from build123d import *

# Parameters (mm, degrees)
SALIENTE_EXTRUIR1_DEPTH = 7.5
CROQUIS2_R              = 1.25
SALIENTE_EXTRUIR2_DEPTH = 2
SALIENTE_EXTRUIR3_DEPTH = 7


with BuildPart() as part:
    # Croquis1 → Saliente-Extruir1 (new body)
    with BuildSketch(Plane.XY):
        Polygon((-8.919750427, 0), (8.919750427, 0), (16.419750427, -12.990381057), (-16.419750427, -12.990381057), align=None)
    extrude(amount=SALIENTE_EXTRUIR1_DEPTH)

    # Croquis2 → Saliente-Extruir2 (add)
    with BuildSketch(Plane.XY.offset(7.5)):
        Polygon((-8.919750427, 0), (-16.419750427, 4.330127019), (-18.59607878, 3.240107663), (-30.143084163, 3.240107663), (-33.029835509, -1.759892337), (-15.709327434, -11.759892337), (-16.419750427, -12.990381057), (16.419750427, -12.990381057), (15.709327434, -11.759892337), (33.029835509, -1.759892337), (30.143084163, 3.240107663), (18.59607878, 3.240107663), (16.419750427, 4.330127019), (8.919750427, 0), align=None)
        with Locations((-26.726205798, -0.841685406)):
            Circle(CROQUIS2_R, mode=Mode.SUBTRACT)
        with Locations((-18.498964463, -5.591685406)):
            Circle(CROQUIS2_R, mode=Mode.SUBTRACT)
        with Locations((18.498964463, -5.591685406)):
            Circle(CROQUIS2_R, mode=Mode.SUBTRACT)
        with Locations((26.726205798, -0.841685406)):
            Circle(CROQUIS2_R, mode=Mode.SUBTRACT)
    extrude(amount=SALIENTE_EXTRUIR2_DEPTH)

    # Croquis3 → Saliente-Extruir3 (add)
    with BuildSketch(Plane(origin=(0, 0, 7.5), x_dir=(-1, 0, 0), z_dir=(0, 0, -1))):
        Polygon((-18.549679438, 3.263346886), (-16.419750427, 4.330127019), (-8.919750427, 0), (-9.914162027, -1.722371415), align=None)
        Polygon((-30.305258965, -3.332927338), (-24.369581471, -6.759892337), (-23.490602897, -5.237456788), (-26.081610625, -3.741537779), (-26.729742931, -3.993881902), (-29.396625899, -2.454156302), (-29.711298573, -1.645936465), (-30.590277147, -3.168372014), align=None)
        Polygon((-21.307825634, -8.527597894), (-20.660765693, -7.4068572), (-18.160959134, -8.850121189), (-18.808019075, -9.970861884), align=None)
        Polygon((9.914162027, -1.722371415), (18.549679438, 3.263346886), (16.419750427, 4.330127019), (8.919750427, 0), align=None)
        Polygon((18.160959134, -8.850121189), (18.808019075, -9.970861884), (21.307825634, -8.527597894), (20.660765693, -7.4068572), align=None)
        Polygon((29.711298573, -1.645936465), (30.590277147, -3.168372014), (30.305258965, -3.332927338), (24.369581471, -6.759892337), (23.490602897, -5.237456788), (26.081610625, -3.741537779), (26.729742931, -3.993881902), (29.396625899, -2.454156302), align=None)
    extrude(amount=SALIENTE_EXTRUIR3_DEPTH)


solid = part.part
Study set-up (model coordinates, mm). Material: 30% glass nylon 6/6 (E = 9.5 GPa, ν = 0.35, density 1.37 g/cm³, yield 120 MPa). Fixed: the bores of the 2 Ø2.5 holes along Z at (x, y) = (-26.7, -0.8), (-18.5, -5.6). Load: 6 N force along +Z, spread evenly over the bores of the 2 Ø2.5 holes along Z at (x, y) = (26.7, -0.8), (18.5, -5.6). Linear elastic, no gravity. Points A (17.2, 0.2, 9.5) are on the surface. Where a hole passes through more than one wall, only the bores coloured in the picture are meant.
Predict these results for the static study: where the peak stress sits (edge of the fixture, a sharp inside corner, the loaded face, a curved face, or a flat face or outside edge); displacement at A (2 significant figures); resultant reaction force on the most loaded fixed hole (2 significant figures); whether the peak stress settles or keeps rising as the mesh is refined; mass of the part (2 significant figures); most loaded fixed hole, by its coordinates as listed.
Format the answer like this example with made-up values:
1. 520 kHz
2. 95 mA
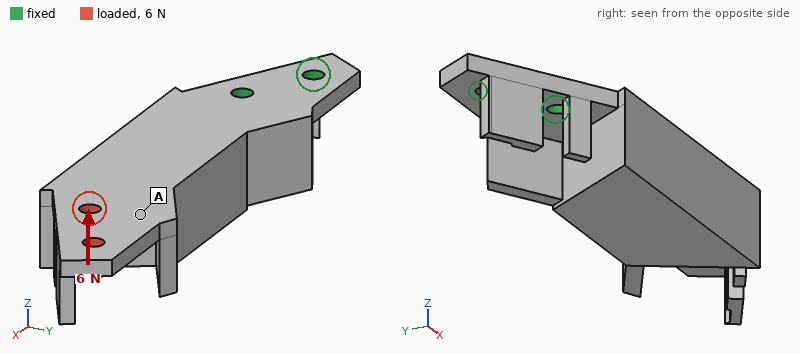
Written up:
1. a sharp inside corner
2. 0.40 mm
3. 18 N
4. keeps rising
5. 6.1 g
6. (-18.5, -5.6)
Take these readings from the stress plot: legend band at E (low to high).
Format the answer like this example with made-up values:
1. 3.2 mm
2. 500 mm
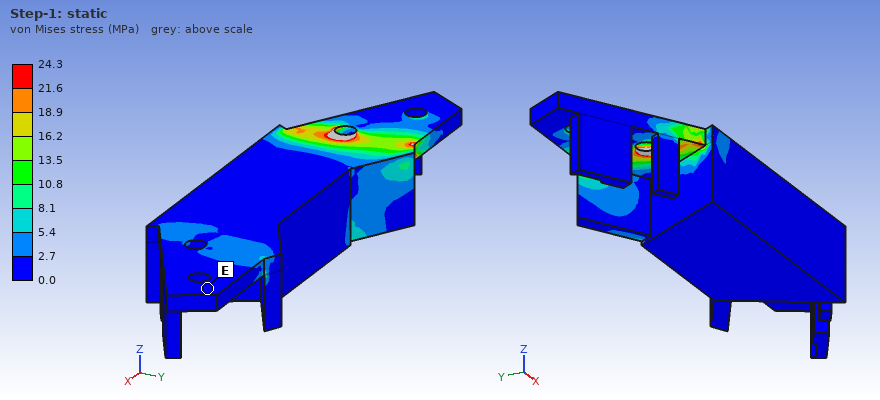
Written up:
1. 0.0 to 2.7 MPa
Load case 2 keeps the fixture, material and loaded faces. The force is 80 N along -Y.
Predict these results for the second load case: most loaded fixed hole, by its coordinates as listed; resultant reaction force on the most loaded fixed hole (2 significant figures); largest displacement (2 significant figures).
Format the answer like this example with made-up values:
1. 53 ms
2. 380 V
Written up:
1. (-18.5, -5.6)
2. 340 N
3. 0.71 mm
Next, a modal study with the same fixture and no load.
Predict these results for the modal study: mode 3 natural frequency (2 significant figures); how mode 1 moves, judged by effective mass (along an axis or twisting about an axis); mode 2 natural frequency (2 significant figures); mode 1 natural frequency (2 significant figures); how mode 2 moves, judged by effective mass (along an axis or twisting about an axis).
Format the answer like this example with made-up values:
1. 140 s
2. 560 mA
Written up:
1. 2400 Hz
2. along Z
3. 1500 Hz
4. 440 Hz
5. along Y
